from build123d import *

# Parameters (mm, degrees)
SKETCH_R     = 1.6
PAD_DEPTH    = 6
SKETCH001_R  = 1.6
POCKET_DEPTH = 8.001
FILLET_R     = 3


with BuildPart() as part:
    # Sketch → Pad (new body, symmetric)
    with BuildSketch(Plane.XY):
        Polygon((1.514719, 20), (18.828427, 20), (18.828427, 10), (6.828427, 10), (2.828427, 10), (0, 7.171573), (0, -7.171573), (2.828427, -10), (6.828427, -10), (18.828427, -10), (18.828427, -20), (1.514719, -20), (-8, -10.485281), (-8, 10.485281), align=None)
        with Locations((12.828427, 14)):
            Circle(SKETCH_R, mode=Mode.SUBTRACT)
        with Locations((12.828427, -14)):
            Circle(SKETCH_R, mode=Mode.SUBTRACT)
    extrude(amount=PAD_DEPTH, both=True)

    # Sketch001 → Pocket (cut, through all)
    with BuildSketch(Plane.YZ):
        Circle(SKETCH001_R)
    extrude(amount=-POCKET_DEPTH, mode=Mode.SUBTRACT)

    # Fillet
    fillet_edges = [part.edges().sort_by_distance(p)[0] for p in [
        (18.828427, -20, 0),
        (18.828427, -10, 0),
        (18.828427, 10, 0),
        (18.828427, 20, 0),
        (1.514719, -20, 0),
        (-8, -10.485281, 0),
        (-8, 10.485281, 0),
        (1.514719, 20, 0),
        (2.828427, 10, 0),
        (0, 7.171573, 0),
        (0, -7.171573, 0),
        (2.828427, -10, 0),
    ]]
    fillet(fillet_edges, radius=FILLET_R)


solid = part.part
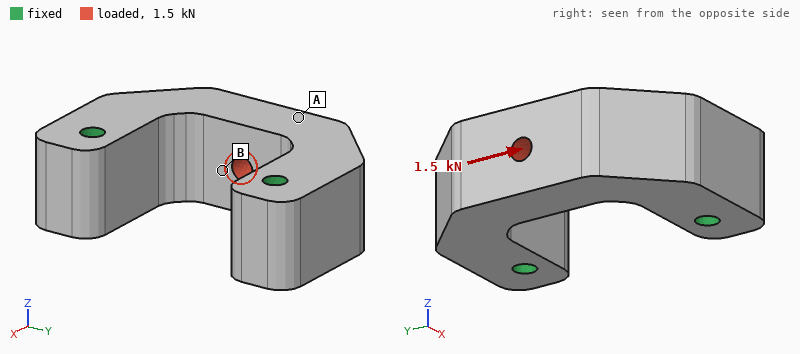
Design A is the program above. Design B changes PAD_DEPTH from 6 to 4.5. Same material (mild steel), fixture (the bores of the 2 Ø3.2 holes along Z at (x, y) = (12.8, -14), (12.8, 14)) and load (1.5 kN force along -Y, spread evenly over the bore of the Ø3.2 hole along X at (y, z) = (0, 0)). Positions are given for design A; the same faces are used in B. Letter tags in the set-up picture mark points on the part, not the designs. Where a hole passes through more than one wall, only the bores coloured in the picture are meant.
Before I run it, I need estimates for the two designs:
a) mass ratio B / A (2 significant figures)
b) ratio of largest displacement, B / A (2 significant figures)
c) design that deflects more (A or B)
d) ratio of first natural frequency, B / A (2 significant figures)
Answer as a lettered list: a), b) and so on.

a) 0.75
b) 1.3
c) B
d) 0.83
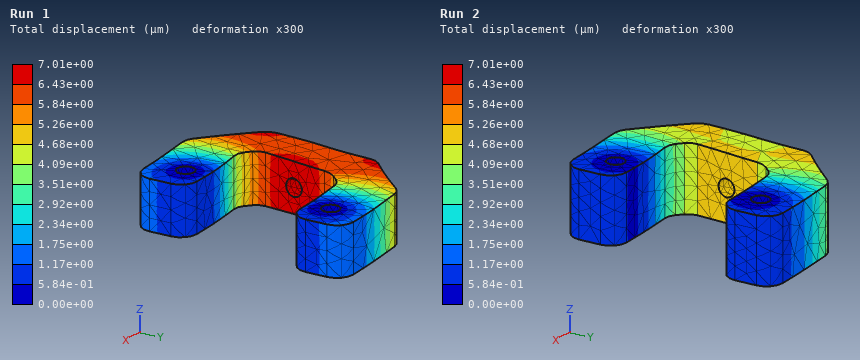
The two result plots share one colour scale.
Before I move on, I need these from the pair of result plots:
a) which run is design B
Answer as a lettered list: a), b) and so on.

a) Run 1
